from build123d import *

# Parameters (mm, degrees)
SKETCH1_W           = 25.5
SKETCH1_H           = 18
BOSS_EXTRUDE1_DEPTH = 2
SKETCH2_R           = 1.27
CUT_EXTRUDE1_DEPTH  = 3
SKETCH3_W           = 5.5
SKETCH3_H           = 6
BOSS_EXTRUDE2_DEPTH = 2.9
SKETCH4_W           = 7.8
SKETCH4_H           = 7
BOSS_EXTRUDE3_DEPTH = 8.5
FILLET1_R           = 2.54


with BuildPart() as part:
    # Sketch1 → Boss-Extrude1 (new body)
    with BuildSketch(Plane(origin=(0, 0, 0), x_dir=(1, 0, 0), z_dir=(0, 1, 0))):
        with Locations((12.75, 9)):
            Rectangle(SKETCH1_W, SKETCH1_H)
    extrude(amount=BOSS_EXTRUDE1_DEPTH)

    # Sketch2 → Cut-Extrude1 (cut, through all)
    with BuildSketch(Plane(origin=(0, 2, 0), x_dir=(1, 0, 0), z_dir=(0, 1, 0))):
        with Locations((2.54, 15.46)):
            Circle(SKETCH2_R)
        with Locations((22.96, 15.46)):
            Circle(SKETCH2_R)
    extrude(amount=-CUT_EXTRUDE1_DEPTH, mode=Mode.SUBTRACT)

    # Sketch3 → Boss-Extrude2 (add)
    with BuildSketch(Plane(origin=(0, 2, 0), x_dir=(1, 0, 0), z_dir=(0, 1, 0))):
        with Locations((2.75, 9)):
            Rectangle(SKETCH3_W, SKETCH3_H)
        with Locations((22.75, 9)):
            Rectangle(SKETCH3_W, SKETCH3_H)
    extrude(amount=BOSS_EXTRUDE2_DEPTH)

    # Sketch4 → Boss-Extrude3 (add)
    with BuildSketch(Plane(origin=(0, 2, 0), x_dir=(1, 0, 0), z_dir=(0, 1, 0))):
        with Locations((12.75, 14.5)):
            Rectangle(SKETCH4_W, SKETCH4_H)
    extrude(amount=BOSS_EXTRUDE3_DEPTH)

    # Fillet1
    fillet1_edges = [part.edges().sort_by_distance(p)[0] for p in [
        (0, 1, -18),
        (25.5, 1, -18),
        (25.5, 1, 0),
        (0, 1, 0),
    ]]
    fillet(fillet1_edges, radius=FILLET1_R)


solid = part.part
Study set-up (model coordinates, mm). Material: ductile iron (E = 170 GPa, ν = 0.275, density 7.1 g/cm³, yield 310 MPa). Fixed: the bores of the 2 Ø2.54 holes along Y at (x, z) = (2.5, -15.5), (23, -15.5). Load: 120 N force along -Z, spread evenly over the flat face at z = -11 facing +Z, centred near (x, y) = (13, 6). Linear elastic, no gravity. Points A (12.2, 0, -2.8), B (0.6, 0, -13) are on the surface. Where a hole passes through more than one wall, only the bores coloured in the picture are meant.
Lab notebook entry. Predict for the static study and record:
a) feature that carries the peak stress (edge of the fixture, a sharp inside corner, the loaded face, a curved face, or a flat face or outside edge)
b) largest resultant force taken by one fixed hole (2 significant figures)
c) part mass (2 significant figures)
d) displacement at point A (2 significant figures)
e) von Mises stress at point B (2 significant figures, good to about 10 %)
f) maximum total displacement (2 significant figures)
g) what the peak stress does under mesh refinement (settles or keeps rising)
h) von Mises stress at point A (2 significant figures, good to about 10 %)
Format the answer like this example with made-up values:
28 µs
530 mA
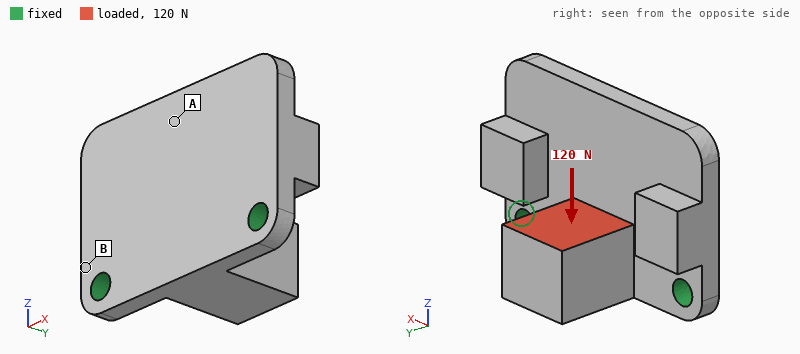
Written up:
edge of the fixture
67 N
11 g
10 µm
32 MPa
12 µm
keeps rising
11 MPa
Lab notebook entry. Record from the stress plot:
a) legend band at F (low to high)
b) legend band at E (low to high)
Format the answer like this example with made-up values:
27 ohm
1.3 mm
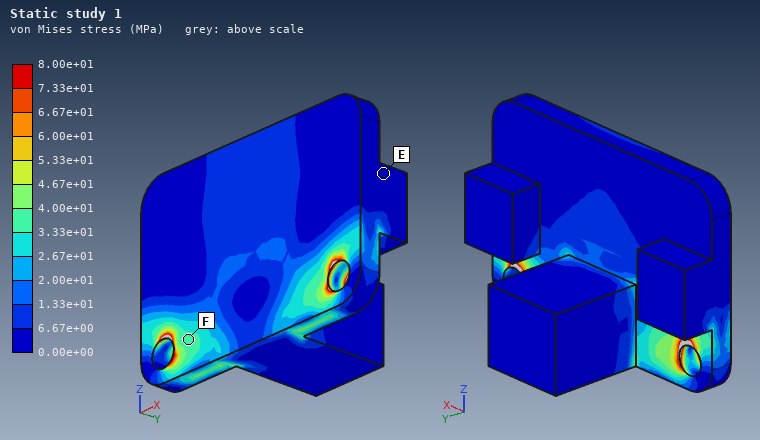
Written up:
3.33e+01 to 4.00e+01 MPa
0.00e+00 to 6.67e+00 MPa
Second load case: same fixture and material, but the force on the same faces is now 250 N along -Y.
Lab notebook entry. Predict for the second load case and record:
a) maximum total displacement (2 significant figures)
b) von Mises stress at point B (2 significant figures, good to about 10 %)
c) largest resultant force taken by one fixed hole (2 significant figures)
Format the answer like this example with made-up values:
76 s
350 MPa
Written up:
23 µm
62 MPa
130 N
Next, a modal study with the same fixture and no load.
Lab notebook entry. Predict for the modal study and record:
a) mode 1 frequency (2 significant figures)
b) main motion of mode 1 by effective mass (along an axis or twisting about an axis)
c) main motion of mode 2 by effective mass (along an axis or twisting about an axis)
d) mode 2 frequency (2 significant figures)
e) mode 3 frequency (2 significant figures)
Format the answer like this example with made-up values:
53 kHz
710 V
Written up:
5600 Hz
along Y
twisting about Z
13 kHz
15 kHz
